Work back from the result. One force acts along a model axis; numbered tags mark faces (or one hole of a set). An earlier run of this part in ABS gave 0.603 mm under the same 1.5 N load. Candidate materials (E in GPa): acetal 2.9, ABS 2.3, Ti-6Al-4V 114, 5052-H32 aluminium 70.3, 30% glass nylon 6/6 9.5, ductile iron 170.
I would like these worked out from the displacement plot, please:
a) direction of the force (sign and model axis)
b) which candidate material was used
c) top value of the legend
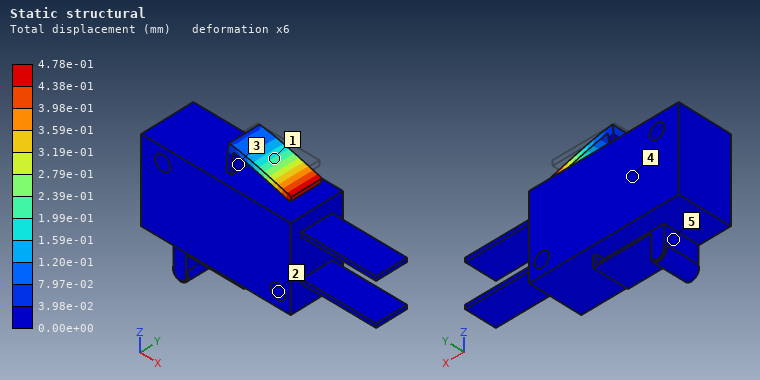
-Z
acetal
4.78e-01 mm
